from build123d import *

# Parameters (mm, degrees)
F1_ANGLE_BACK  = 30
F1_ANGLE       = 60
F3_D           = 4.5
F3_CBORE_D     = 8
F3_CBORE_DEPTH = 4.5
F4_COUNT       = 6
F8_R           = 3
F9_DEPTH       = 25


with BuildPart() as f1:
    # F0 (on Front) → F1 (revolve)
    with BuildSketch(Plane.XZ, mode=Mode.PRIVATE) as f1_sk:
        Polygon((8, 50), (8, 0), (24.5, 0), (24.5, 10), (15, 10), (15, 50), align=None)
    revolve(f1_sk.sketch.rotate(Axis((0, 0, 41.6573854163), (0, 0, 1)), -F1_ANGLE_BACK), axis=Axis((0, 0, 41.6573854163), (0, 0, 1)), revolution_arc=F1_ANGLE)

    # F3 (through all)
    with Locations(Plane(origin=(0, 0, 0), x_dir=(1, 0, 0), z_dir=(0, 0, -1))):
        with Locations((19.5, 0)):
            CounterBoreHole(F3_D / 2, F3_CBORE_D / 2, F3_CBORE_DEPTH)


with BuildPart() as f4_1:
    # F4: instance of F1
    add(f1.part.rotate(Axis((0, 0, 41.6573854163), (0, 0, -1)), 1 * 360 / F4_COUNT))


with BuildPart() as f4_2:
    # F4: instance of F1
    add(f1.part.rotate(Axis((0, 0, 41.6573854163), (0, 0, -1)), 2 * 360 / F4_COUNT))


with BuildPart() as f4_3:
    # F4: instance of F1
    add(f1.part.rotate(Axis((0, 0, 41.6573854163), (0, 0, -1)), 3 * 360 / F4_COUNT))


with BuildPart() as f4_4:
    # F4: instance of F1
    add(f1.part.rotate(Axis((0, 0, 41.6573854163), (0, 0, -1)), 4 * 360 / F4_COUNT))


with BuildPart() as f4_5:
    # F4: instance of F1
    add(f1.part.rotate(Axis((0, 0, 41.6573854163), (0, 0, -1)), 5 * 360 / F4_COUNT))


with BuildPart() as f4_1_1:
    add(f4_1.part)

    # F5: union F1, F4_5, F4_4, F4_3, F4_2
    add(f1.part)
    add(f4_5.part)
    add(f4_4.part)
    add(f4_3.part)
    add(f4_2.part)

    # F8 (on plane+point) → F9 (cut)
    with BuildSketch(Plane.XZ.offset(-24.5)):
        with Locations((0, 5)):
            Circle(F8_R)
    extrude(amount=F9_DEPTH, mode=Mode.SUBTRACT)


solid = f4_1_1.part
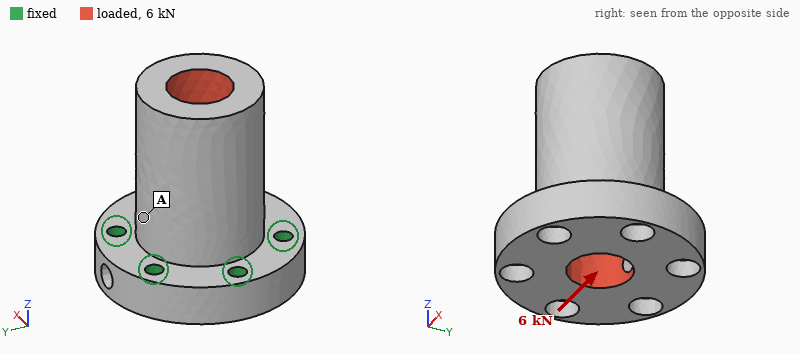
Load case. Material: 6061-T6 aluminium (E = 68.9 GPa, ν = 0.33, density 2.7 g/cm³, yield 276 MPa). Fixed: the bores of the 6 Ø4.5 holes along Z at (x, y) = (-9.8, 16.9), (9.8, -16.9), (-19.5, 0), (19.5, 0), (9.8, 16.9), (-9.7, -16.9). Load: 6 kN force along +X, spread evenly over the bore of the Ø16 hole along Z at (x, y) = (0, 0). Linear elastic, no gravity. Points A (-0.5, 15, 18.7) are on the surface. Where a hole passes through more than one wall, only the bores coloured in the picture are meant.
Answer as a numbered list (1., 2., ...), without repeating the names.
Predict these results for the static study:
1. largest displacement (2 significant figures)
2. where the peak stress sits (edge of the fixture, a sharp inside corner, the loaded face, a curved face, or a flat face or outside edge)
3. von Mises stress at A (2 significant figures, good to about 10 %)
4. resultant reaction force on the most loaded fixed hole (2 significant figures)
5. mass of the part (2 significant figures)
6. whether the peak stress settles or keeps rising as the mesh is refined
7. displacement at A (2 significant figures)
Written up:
1. 48 µm
2. edge of the fixture
3. 14 MPa
4. 2.4 kN
5. 94 g
6. keeps rising
7. 10 µm
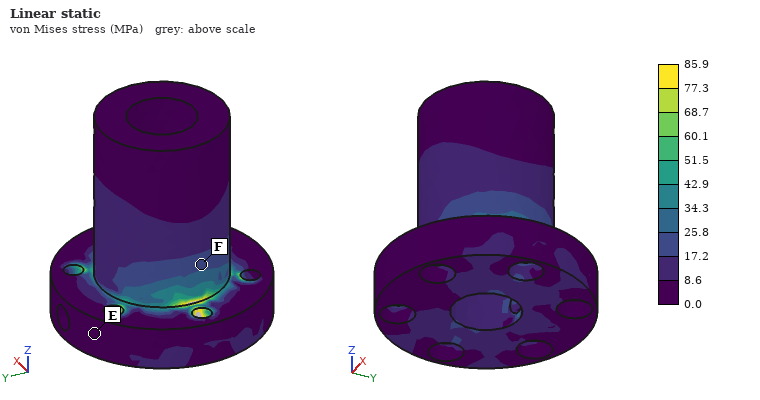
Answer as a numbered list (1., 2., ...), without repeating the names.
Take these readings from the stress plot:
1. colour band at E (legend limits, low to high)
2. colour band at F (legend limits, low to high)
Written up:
1. 0.0 to 8.6 MPa
2. 17.2 to 25.8 MPa
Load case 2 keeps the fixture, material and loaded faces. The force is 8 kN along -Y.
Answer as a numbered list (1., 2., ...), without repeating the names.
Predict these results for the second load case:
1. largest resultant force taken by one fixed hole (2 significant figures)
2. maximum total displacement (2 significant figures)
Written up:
1. 2.8 kN
2. 65 µm
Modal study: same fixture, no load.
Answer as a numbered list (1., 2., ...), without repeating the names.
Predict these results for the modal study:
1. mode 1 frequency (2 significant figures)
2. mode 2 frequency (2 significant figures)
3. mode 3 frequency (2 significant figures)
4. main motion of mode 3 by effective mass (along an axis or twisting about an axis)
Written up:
1. 8100 Hz
2. 8100 Hz
3. 18 kHz
4. twisting about Z
